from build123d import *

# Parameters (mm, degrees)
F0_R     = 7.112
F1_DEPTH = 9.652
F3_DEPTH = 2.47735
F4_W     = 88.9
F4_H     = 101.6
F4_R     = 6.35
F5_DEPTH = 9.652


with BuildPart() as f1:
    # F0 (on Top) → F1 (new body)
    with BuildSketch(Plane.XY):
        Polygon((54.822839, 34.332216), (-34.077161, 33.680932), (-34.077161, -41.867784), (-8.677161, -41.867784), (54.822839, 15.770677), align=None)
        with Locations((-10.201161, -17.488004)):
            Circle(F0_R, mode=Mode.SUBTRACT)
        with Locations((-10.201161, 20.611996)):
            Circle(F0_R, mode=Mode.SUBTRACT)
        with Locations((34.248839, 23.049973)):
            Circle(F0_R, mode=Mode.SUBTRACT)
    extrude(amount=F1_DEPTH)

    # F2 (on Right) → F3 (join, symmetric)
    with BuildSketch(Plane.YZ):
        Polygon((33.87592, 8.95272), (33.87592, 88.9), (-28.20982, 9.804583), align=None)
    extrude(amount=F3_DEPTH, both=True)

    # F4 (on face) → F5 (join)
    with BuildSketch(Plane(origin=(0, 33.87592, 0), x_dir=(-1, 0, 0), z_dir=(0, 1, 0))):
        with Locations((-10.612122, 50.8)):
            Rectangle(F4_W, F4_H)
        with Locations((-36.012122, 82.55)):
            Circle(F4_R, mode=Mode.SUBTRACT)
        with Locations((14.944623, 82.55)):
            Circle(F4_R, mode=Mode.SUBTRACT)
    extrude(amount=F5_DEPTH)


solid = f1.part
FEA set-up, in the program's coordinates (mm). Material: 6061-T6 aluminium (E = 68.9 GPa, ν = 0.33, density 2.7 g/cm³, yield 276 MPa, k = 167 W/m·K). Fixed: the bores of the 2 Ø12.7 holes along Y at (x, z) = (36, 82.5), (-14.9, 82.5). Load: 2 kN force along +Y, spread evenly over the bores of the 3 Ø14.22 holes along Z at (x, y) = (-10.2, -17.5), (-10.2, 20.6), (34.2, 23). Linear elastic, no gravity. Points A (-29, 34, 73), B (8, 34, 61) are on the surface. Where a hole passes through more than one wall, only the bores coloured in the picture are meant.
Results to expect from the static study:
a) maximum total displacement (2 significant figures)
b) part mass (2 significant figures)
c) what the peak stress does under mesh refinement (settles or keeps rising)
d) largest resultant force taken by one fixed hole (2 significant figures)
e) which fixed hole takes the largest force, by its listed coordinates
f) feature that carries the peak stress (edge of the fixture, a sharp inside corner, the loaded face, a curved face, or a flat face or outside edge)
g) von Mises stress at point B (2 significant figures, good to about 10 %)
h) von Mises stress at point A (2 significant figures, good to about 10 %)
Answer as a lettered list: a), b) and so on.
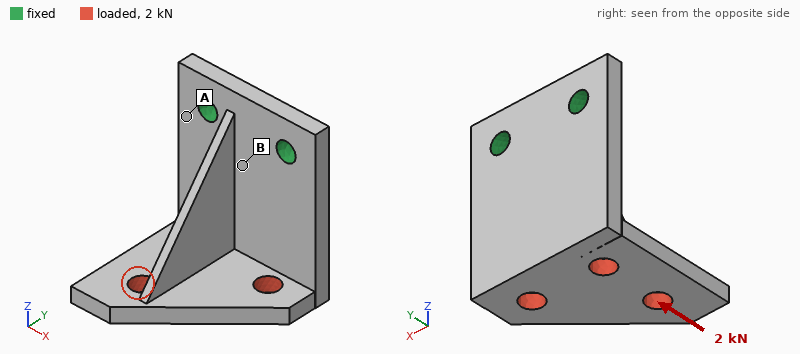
a) 0.59 mm
b) 380 g
c) keeps rising
d) 1.1 kN
e) (-14.9, 82.5)
f) edge of the fixture
g) 27 MPa
h) 61 MPa
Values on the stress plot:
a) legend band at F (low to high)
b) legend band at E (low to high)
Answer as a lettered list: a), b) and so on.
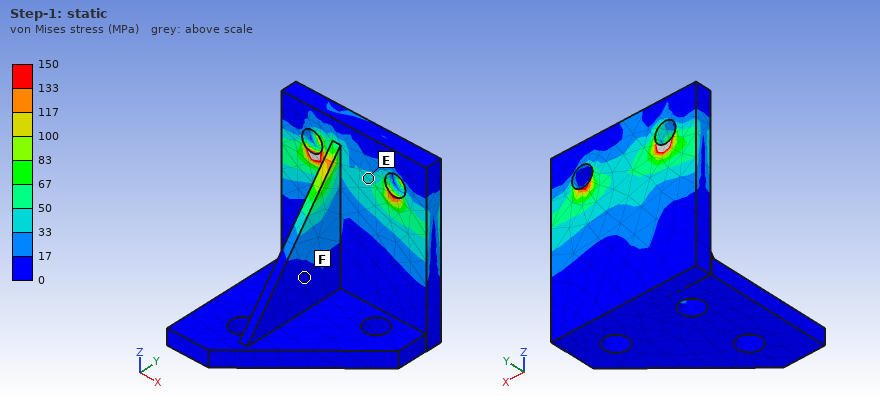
a) 0 to 17 MPa
b) 33 to 50 MPa
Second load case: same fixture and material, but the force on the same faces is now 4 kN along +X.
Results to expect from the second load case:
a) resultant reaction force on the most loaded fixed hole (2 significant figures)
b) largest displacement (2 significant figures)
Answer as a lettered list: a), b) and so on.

a) 5.9 kN
b) 0.79 mm
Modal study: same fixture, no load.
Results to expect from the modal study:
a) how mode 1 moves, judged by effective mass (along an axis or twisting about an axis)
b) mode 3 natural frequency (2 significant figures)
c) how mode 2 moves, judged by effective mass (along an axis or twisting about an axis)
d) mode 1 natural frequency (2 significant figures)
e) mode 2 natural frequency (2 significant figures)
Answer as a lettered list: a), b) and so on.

a) along Y
b) 2800 Hz
c) along X
d) 760 Hz
e) 1100 Hz
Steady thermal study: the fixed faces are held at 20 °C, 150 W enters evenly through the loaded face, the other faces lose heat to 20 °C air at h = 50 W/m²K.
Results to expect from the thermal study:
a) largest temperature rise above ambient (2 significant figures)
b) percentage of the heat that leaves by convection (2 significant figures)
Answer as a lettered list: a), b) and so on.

a) 75 K
b) 42 %
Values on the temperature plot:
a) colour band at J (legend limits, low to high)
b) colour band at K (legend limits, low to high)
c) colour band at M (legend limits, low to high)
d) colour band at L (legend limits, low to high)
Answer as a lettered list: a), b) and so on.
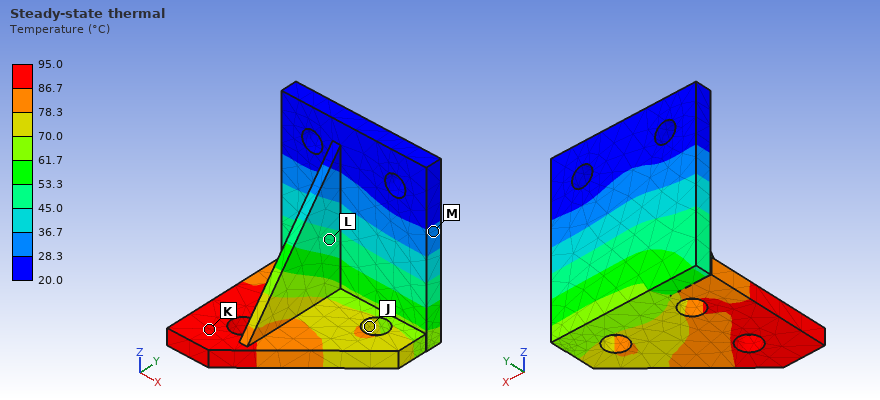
a) 70.0 to 78.3 °C
b) 86.7 to 95.0 °C
c) 28.3 to 36.7 °C
d) 45.0 to 53.3 °C
